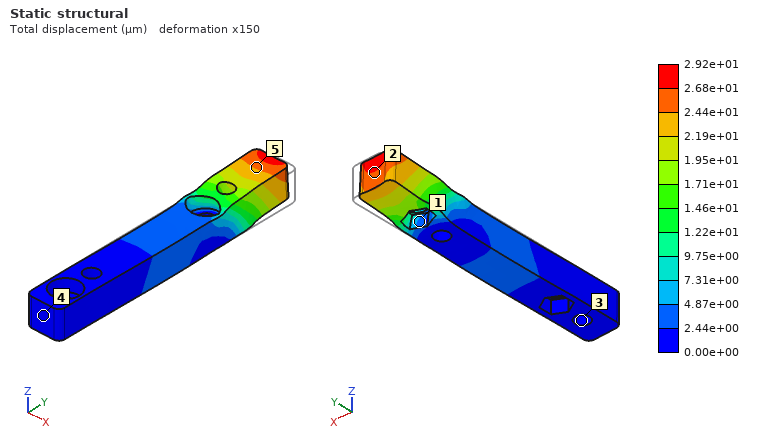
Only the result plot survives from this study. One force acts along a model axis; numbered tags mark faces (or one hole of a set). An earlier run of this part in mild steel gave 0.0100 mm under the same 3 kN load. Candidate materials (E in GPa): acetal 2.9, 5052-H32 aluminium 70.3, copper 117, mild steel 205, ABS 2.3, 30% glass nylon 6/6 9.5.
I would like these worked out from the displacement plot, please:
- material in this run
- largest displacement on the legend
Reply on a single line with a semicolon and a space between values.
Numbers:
5052-H32 aluminium; 2.92e+01 µm
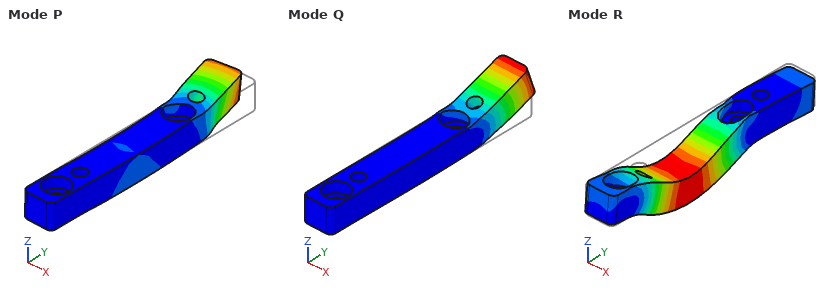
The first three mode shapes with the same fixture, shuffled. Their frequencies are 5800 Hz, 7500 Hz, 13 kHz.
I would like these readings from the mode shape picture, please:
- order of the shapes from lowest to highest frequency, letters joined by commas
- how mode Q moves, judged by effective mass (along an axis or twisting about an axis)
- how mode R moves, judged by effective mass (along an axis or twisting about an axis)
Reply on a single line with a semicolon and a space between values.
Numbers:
Q, P, R; along Z; along Z
